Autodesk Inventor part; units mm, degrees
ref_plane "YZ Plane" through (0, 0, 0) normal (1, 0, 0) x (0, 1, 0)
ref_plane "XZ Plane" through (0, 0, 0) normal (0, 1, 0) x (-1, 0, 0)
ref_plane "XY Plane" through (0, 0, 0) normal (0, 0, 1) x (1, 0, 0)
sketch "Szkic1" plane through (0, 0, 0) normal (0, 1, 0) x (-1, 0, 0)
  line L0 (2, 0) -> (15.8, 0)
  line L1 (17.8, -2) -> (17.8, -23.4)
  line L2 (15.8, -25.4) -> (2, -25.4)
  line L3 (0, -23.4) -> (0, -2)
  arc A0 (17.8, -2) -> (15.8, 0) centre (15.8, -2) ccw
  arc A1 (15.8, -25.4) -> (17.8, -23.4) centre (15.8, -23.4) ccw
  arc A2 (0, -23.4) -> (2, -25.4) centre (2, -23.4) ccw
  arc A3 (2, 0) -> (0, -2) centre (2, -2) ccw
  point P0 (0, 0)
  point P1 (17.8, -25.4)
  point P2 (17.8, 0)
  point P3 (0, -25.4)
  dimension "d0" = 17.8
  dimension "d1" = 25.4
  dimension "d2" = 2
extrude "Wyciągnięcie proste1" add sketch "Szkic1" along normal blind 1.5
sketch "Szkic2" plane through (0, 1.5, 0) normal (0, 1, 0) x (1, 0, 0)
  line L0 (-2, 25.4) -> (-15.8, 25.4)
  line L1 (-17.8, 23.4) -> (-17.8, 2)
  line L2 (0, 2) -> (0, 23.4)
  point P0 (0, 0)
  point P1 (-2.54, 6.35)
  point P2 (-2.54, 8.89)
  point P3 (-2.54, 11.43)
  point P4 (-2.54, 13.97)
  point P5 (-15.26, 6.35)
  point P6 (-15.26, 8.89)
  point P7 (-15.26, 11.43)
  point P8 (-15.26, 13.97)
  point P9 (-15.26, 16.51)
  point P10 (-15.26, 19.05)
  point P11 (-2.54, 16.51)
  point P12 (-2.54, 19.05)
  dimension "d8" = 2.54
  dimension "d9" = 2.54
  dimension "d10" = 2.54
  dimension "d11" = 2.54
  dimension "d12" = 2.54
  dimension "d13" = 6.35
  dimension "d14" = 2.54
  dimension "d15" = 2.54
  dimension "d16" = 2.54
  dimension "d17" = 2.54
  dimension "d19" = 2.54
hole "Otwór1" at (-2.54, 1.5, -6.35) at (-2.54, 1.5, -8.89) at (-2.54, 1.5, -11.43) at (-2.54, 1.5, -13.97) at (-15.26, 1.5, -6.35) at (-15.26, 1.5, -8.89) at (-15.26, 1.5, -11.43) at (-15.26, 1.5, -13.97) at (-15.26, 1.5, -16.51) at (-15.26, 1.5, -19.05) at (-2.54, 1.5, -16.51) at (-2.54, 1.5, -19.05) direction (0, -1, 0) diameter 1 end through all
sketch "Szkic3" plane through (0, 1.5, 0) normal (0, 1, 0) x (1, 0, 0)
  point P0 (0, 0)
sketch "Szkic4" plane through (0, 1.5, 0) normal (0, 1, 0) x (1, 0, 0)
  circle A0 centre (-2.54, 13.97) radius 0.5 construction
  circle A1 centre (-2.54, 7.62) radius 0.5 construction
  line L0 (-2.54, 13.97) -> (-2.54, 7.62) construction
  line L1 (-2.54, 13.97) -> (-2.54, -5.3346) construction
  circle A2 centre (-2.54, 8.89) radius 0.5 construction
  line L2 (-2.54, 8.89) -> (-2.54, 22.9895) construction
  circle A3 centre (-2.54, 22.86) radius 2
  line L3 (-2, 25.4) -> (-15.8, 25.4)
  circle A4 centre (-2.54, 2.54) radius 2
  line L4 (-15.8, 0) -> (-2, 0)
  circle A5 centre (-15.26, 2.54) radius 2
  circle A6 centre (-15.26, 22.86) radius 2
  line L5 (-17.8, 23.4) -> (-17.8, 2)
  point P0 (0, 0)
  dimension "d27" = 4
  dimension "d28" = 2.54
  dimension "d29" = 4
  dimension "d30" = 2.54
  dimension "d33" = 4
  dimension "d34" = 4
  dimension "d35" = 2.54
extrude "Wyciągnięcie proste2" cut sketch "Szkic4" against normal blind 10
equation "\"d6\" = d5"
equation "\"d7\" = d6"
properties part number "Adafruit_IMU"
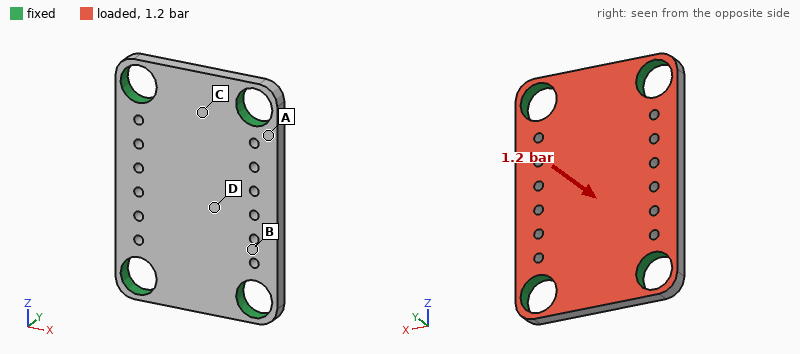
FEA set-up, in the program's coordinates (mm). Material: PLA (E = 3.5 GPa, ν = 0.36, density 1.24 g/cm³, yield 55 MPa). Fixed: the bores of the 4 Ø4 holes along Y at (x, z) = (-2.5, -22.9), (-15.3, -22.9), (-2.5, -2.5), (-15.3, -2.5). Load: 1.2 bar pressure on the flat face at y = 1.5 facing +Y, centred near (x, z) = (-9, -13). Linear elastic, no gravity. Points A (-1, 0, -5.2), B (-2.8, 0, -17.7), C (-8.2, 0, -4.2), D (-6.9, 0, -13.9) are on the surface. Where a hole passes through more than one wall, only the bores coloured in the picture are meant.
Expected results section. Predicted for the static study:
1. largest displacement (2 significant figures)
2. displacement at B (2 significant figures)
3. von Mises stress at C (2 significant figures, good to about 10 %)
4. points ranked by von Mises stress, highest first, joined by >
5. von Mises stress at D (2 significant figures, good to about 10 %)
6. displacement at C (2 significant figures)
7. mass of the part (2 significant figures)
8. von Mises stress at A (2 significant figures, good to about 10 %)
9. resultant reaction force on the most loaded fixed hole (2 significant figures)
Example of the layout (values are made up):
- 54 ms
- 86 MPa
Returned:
- 37 µm
- 16 µm
- 2.6 MPa
- A > D > C > B
- 3.6 MPa
- 8.2 µm
- 0.72 g
- 5.3 MPa
- 12 N
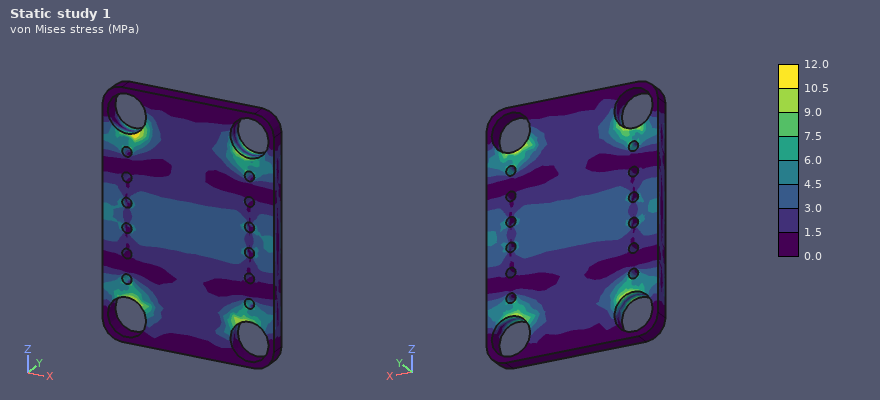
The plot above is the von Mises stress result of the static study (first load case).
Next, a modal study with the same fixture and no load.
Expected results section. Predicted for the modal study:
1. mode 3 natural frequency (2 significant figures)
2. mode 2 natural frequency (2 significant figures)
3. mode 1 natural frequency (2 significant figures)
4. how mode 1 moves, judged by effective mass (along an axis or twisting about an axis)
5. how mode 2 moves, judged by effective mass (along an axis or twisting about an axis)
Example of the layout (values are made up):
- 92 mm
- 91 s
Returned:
- 14 kHz
- 9900 Hz
- 7700 Hz
- along Y
- twisting about Z
